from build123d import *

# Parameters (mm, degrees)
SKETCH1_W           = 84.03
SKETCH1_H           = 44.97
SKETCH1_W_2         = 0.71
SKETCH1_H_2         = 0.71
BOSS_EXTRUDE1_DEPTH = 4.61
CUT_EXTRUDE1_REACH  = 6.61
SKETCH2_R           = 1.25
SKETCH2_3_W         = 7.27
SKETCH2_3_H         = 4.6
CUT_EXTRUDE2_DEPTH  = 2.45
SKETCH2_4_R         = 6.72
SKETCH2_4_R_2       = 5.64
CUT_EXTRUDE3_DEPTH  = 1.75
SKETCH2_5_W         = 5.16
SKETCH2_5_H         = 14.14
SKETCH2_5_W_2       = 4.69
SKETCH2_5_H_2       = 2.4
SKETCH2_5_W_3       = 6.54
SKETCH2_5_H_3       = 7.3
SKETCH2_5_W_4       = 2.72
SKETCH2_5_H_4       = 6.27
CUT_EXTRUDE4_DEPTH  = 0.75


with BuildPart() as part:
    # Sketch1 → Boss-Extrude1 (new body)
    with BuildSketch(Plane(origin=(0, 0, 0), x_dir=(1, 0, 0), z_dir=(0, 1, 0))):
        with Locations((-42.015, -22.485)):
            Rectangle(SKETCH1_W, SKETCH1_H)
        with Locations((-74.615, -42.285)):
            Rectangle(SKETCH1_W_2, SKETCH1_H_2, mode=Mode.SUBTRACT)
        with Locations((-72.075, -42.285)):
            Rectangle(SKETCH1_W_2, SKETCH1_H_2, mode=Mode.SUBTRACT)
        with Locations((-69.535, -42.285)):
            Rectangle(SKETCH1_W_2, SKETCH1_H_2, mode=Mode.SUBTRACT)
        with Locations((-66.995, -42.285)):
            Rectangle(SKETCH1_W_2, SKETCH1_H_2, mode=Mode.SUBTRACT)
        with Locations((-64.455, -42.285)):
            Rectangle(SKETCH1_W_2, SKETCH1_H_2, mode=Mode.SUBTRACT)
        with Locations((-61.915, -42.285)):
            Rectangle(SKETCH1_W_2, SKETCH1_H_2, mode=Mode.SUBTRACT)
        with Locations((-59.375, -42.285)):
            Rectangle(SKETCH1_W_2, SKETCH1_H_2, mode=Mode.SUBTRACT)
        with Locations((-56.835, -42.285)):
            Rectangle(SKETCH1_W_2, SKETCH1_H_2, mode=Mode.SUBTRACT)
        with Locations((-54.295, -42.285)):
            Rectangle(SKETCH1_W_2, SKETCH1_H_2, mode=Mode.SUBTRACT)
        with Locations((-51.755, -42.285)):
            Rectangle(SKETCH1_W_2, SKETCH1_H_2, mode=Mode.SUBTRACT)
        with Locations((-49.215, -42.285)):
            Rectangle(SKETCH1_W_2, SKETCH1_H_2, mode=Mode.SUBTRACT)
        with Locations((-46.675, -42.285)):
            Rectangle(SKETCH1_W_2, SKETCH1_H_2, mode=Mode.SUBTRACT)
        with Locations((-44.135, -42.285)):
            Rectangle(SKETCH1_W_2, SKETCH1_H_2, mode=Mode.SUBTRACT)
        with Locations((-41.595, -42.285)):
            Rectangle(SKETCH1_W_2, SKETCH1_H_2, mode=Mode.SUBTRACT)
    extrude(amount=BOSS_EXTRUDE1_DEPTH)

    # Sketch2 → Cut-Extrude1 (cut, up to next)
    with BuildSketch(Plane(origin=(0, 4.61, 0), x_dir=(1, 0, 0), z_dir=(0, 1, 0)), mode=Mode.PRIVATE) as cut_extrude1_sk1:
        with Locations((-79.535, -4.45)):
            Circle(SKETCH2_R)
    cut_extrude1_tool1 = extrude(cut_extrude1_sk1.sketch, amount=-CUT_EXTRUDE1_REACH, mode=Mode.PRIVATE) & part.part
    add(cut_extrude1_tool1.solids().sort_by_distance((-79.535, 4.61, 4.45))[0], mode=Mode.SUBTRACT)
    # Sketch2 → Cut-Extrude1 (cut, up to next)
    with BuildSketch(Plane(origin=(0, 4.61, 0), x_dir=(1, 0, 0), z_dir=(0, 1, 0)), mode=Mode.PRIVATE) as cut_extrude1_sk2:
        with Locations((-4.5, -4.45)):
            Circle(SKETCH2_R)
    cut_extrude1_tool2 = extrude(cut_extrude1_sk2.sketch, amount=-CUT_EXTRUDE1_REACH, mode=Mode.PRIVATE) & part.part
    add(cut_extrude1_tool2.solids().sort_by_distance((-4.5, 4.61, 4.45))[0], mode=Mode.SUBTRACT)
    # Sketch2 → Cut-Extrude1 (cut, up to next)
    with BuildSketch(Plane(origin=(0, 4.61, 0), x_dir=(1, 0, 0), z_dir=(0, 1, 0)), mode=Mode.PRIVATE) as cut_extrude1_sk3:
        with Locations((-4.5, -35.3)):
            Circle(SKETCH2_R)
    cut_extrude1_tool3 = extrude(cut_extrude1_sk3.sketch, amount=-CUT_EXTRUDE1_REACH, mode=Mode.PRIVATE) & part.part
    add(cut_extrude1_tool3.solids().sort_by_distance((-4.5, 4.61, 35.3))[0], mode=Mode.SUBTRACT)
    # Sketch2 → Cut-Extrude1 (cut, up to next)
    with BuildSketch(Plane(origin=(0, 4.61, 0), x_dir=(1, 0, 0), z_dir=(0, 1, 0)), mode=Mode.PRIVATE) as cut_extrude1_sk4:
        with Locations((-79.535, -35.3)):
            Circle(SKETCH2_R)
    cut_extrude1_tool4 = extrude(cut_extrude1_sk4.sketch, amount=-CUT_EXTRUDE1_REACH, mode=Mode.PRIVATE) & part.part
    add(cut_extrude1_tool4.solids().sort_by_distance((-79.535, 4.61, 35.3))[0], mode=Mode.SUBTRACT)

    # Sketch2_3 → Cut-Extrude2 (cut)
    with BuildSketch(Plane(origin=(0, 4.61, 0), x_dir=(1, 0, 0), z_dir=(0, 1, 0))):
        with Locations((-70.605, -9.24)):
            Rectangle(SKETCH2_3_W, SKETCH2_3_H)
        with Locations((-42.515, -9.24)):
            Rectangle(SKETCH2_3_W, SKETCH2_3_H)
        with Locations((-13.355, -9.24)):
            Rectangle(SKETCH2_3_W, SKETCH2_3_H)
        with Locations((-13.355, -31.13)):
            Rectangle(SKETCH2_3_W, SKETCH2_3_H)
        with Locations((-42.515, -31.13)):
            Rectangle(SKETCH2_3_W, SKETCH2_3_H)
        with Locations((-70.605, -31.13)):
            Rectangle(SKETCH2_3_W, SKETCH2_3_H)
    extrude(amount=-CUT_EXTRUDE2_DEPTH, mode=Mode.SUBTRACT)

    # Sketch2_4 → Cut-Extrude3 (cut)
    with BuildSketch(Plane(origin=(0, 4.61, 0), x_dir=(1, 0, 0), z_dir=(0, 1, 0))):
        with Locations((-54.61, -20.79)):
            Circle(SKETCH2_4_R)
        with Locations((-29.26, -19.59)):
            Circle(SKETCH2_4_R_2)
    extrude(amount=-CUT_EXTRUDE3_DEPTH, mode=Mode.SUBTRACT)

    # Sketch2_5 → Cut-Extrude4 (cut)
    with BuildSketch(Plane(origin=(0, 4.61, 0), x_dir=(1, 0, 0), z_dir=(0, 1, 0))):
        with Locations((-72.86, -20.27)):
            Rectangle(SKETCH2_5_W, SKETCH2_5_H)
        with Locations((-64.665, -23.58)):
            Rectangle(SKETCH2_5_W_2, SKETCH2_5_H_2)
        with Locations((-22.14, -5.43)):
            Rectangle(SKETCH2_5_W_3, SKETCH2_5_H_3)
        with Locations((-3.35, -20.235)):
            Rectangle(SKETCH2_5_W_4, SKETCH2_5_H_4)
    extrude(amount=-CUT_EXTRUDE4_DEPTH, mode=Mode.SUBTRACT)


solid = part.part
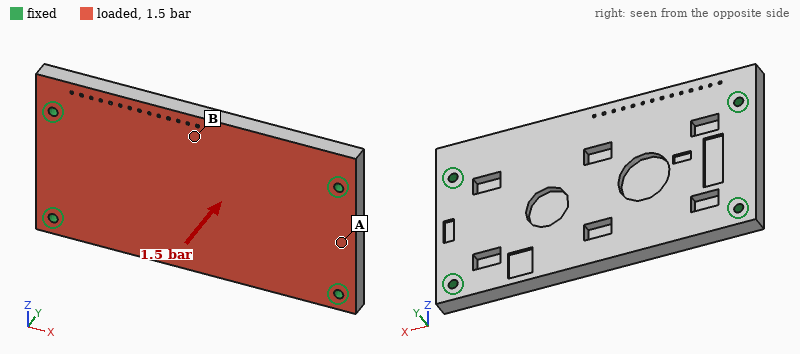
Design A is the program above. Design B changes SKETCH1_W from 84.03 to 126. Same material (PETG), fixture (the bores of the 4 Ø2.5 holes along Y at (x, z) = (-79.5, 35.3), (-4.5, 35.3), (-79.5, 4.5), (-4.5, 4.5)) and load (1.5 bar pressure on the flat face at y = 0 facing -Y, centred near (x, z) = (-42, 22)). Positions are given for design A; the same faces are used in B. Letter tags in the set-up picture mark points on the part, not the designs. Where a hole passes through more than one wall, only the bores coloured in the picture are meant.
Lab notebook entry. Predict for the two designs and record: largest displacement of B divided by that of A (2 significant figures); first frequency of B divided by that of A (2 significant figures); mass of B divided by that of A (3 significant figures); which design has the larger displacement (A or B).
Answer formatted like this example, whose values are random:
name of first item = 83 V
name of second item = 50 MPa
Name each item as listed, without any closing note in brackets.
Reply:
largest displacement of B divided by that of A = 0.83
first frequency of B divided by that of A = 0.97
mass of B divided by that of A = 1.53
which design has the larger displacement = A
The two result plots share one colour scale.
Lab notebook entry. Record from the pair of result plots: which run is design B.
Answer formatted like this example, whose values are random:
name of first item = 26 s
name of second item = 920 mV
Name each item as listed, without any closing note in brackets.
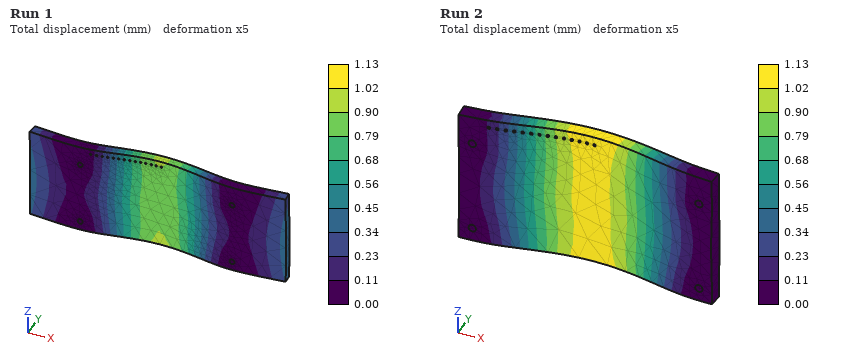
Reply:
which run is design B = Run 1
